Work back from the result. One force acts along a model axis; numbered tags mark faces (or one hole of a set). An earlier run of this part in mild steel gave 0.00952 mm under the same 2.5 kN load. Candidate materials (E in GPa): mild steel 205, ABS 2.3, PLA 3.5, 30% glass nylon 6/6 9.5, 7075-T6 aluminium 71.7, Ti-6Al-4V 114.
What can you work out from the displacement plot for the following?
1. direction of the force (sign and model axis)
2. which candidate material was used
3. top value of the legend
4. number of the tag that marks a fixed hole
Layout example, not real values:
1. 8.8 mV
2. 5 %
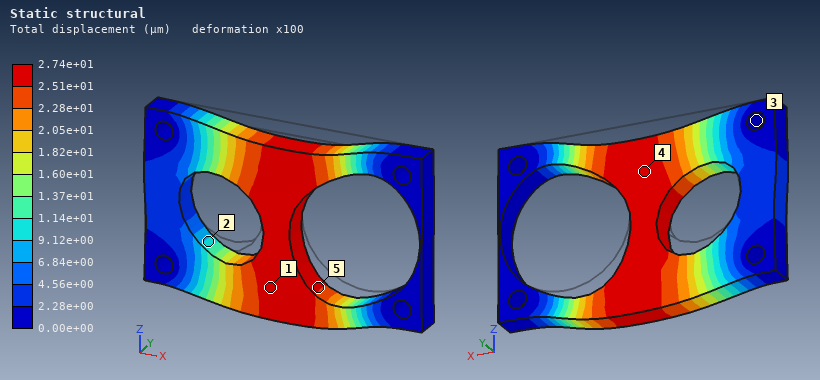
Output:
1. -Z
2. 7075-T6 aluminium
3. 2.74e+01 µm
4. 3
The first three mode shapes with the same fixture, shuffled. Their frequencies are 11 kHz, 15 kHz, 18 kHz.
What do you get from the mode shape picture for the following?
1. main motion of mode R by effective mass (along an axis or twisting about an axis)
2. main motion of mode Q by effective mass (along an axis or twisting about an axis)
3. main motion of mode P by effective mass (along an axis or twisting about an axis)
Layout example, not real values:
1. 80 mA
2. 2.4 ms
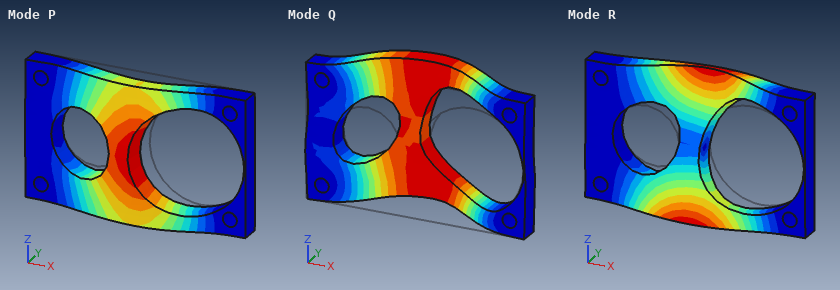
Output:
1. twisting about X
2. along Z
3. along Y
